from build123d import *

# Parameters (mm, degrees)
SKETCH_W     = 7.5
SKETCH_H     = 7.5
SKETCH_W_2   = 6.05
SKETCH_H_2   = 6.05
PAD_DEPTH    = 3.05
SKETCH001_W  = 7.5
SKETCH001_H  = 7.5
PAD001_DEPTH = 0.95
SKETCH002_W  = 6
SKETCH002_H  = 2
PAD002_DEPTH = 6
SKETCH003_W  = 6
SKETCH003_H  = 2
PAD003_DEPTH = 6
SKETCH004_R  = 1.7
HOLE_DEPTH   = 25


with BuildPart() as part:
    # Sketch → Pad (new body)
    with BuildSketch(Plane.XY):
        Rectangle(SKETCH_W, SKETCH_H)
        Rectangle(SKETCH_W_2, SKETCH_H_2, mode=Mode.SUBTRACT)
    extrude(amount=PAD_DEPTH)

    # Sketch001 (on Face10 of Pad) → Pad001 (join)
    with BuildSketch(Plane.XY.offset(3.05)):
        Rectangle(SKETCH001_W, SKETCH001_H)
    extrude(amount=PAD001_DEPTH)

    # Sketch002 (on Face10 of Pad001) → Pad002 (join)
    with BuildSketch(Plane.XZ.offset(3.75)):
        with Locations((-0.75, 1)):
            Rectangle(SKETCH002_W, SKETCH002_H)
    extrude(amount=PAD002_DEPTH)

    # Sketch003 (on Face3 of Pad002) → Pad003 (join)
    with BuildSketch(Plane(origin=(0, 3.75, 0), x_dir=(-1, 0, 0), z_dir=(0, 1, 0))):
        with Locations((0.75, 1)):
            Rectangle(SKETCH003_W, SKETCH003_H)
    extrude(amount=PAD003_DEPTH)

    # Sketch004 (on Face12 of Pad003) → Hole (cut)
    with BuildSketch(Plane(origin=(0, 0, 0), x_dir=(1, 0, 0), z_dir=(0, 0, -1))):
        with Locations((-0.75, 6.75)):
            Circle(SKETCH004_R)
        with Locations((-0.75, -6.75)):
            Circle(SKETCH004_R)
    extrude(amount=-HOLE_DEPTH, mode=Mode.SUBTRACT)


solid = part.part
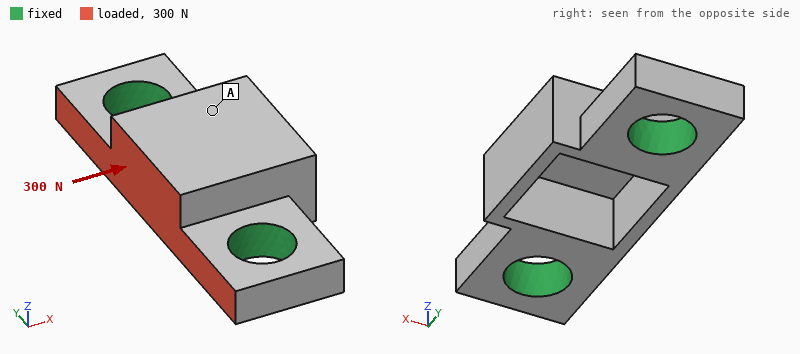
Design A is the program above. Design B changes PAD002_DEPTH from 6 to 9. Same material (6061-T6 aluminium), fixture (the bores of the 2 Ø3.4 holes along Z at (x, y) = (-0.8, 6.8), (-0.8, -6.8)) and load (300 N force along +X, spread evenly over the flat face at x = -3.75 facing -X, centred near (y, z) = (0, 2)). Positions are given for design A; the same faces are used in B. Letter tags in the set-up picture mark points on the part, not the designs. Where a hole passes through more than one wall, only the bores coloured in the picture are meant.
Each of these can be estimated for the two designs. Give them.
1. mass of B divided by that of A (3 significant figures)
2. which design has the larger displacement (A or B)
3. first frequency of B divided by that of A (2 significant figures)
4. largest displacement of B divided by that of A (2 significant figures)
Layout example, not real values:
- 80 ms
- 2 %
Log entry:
- 1.16
- A
- 1.00
- 0.90
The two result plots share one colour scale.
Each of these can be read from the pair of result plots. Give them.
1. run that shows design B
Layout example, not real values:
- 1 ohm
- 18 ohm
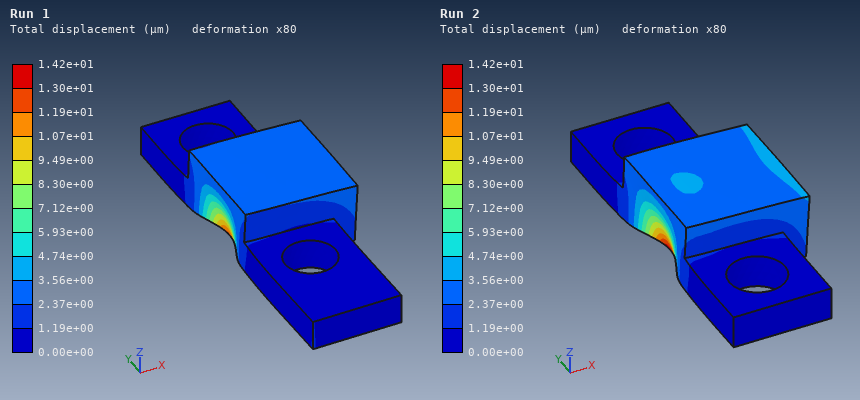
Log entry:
- Run 1
